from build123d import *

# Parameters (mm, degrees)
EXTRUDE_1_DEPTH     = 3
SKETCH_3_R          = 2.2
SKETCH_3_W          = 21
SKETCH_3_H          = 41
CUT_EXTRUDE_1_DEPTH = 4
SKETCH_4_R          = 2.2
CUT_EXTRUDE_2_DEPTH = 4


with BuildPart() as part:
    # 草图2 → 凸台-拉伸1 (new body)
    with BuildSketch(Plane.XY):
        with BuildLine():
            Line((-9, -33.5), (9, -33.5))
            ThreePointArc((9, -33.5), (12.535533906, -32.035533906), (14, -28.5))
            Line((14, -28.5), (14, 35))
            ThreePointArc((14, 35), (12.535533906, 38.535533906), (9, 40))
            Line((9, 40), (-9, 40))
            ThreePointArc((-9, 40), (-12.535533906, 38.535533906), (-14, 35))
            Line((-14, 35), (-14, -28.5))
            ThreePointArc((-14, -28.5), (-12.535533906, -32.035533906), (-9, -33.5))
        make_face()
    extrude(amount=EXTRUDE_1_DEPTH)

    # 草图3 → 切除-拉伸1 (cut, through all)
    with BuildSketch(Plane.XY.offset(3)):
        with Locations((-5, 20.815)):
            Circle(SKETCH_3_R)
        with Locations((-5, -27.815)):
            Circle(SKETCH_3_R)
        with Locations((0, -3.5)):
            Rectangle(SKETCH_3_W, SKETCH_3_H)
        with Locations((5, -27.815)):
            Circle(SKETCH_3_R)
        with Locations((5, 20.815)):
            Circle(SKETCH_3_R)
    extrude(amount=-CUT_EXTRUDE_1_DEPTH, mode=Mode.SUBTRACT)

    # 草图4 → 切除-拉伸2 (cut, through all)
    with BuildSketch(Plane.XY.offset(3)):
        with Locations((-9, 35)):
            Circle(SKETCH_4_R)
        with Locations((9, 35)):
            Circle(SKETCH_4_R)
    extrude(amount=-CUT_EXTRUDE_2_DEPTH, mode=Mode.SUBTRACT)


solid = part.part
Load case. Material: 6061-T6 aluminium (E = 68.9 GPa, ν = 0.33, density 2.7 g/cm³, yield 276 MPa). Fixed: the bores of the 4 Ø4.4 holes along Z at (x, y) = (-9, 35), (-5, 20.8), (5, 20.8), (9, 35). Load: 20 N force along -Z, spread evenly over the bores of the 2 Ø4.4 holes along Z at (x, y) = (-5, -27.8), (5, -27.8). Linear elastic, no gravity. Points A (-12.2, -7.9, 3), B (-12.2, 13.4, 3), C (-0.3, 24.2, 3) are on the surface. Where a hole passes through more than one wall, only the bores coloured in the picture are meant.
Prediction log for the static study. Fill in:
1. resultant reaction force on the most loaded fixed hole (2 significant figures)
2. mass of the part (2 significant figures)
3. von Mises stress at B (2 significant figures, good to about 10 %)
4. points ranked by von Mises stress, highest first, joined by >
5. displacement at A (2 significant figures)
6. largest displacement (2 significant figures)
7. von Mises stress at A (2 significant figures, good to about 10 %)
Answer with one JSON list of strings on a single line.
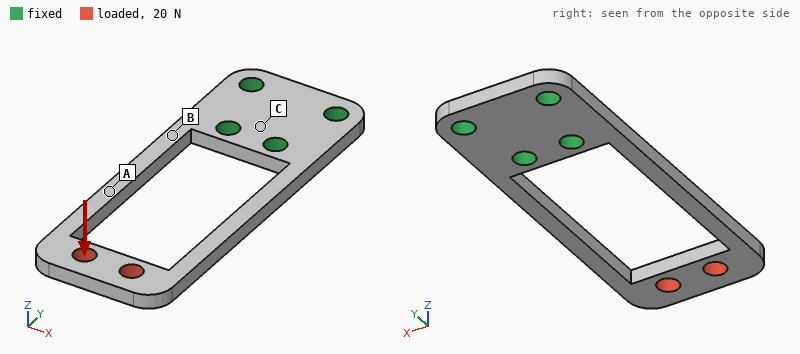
["29 N", "8.8 g", "79 MPa", "B > A > C", "0.29 mm", "0.82 mm", "38 MPa"]
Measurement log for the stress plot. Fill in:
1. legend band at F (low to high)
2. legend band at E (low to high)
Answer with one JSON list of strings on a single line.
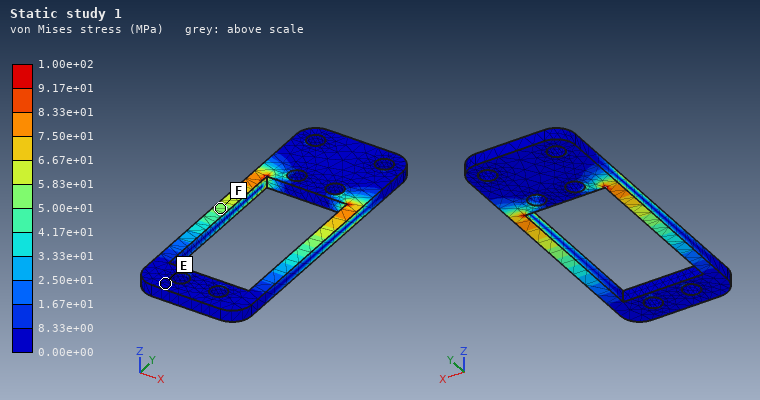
["5.00e+01 to 5.83e+01 MPa", "0.00e+00 to 8.33e+00 MPa"]
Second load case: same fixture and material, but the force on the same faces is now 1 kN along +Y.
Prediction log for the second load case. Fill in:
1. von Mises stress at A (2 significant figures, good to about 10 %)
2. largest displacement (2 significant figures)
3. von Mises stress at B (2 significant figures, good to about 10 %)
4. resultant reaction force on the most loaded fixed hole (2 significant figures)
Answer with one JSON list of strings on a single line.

["48 MPa", "64 µm", "47 MPa", "280 N"]
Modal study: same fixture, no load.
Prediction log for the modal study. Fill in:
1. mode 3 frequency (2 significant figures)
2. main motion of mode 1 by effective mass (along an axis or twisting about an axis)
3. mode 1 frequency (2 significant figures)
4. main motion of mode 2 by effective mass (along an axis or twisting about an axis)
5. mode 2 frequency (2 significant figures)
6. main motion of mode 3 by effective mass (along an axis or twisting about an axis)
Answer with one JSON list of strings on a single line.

["1800 Hz", "along Z", "550 Hz", "along X", "1300 Hz", "twisting about Y"]
